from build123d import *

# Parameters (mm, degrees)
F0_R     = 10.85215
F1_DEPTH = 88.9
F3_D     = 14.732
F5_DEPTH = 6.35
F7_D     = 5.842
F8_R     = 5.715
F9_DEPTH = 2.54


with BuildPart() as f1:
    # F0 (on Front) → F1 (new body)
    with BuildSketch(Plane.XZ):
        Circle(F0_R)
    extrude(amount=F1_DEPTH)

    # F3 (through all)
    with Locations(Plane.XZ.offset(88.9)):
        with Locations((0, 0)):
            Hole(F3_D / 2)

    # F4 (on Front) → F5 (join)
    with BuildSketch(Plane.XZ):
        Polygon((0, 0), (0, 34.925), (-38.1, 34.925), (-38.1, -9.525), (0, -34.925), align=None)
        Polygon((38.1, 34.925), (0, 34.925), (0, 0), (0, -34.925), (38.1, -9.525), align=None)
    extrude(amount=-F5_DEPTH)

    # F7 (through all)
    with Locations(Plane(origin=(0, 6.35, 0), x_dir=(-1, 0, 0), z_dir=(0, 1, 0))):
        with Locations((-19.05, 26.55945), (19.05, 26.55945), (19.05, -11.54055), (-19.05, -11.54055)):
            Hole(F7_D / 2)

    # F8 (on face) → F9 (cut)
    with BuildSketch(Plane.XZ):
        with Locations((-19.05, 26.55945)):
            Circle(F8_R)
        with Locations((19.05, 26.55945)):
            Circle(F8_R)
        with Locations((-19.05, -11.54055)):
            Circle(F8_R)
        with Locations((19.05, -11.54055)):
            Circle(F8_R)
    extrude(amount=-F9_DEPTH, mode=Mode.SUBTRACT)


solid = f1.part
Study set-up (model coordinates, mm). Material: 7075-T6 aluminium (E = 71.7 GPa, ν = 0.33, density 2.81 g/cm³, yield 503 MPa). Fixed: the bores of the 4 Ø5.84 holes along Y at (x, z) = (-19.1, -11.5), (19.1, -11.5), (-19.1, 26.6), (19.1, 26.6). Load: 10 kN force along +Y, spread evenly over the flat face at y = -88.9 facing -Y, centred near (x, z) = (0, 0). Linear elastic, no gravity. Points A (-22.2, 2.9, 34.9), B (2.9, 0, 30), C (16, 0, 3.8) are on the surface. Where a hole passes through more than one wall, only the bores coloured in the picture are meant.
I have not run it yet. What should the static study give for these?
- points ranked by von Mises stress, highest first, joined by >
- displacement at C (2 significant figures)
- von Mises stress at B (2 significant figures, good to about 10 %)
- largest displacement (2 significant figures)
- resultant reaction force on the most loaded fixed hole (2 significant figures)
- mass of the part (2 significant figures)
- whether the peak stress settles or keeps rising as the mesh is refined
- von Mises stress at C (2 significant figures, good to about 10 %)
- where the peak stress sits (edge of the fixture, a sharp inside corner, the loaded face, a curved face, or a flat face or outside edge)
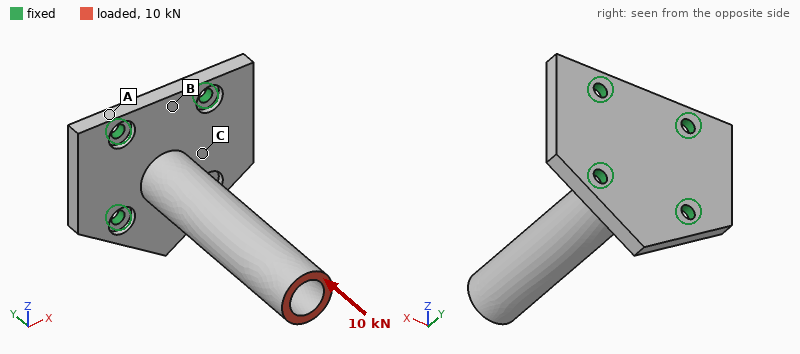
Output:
C > B > A
0.041 mm
33 MPa
0.16 mm
4.3 kN
120 g
keeps rising
66 MPa
edge of the fixture
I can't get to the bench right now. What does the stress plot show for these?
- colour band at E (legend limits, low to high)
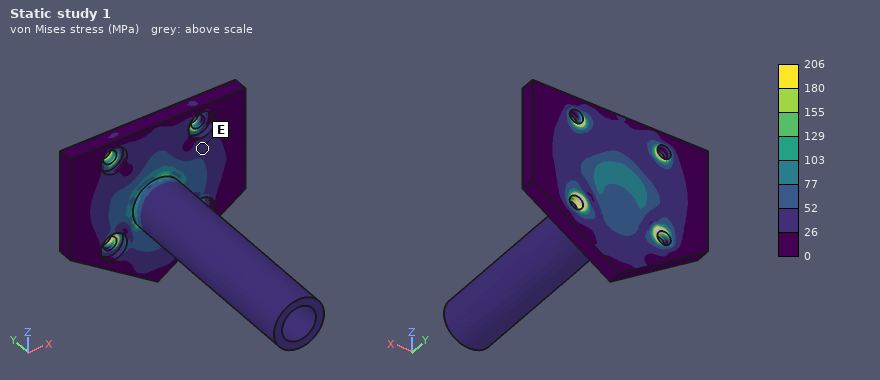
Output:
26 to 52 MPa
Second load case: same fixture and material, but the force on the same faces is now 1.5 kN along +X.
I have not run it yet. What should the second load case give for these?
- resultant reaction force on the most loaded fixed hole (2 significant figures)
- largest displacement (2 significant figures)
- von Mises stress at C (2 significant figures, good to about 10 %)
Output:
3.4 kN
0.96 mm
69 MPa
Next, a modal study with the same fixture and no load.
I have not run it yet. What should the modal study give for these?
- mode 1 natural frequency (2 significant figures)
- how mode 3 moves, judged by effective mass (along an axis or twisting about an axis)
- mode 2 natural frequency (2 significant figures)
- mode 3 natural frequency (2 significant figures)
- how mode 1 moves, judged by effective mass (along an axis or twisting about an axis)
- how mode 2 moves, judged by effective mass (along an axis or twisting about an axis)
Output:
1600 Hz
along Y
1700 Hz
7200 Hz
along Z
along X
